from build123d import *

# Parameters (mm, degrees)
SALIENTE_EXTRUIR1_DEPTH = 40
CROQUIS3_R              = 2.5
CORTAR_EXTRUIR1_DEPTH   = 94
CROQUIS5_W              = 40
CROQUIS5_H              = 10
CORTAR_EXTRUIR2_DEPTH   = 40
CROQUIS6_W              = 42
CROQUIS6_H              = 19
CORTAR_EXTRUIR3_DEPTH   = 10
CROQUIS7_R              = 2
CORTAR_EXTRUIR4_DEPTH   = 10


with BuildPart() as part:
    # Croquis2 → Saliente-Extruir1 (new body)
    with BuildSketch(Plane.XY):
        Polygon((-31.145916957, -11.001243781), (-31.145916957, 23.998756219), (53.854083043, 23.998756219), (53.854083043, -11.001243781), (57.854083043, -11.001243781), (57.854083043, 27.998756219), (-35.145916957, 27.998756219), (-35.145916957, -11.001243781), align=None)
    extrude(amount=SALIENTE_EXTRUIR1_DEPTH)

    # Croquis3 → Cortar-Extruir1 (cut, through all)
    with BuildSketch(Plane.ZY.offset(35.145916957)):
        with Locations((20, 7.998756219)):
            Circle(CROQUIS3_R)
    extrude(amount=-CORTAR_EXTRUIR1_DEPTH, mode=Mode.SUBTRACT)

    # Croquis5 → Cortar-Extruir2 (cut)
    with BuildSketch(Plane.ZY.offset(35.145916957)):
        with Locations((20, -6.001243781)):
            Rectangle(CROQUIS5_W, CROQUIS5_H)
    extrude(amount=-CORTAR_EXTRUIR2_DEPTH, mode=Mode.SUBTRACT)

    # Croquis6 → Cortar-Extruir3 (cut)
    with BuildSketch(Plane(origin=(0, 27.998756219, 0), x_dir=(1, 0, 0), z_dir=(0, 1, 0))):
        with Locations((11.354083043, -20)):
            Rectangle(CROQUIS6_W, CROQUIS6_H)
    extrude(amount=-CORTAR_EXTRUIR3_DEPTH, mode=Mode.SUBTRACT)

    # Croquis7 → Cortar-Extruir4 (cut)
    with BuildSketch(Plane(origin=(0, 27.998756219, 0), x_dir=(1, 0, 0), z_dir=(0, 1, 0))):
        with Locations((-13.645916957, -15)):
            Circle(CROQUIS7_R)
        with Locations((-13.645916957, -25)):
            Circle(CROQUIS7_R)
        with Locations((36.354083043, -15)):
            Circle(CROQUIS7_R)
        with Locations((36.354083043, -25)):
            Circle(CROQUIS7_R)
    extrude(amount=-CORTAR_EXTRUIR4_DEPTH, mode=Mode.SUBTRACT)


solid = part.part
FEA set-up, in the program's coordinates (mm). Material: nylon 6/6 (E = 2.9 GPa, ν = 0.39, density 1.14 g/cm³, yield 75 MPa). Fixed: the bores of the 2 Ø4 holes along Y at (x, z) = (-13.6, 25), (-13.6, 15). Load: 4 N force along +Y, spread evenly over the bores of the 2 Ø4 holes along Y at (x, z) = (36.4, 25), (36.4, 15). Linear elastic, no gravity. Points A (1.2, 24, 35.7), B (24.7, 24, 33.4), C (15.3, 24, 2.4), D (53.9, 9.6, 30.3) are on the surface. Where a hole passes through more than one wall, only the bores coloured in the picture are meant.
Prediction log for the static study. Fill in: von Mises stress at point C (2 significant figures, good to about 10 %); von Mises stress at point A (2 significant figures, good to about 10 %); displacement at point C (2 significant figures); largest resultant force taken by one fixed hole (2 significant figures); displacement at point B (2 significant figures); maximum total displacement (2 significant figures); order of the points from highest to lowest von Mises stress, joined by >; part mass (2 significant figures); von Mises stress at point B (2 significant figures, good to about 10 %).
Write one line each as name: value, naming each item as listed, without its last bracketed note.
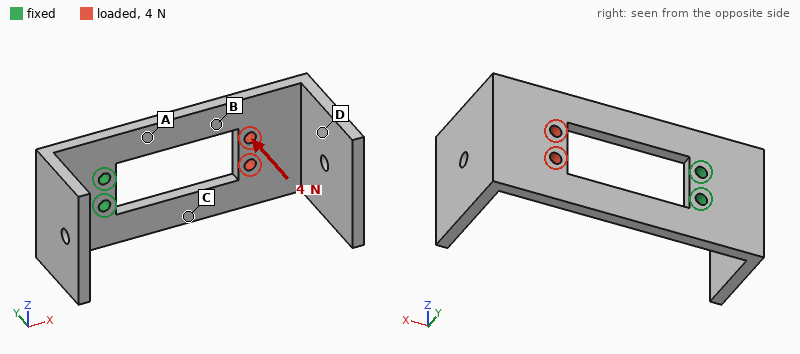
von Mises stress at point C: 1.5 MPa
von Mises stress at point A: 2.5 MPa
displacement at point C: 0.27 mm
largest resultant force taken by one fixed hole: 2.0 N
displacement at point B: 0.41 mm
maximum total displacement: 1.2 mm
order of the points from highest to lowest von Mises stress, joined by >: A > C > B > D
part mass: 24 g
von Mises stress at point B: 0.86 MPa
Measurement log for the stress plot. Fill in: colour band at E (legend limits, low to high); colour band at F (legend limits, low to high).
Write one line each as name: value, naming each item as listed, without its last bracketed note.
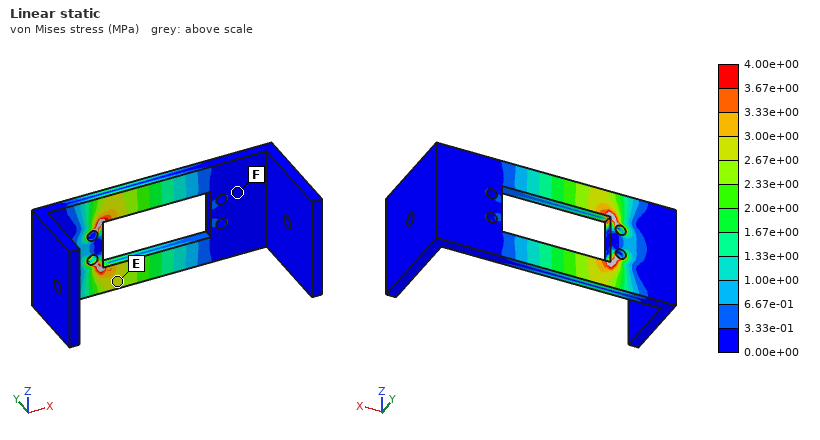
colour band at E: 2.67e+00 to 3.00e+00 MPa
colour band at F: 0.00e+00 to 3.33e-01 MPa
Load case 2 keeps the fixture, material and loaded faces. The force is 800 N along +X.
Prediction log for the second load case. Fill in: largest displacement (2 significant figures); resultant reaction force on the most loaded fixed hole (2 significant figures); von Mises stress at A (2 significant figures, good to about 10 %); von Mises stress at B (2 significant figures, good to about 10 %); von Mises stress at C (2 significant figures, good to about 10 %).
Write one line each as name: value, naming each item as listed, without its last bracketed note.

largest displacement: 0.32 mm
resultant reaction force on the most loaded fixed hole: 420 N
von Mises stress at A: 8.9 MPa
von Mises stress at B: 11 MPa
von Mises stress at C: 7.4 MPa
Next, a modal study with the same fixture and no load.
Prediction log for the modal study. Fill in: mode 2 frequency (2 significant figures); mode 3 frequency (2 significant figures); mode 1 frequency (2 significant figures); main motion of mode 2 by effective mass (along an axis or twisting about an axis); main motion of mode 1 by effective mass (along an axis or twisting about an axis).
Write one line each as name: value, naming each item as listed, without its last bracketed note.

mode 2 frequency: 200 Hz
mode 3 frequency: 390 Hz
mode 1 frequency: 78 Hz
main motion of mode 2 by effective mass: along Z
main motion of mode 1 by effective mass: along Y
